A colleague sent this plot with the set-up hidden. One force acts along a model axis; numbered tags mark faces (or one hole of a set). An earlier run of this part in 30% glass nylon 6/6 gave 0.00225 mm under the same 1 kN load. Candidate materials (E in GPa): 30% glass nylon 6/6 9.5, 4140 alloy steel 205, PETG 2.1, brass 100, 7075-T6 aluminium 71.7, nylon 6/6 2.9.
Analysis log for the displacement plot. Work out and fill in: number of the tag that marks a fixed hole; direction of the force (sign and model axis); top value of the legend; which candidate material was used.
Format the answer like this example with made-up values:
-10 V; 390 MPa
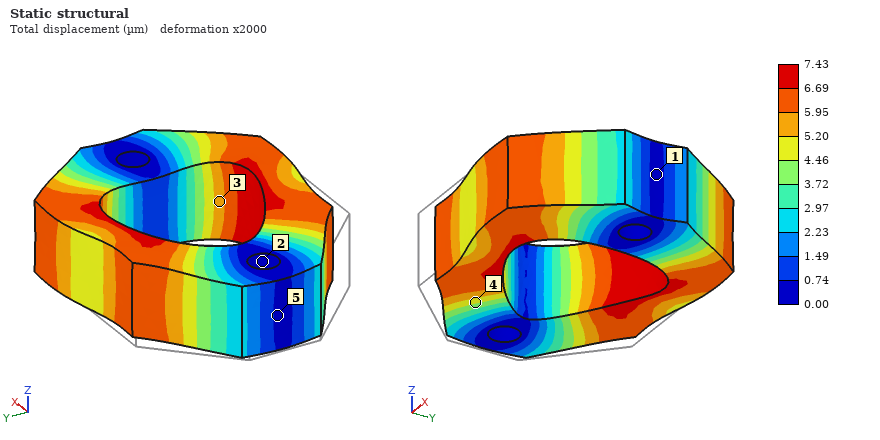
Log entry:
2; +X; 7.43 µm; nylon 6/6
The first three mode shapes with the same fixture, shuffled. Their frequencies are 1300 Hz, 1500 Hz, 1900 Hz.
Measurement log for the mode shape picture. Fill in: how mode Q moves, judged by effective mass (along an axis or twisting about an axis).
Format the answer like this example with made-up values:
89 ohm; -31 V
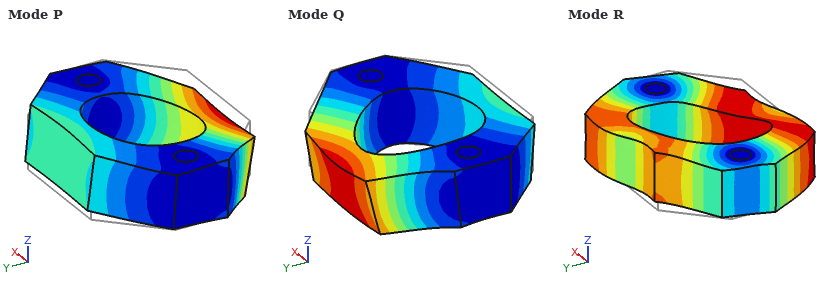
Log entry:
along Z
